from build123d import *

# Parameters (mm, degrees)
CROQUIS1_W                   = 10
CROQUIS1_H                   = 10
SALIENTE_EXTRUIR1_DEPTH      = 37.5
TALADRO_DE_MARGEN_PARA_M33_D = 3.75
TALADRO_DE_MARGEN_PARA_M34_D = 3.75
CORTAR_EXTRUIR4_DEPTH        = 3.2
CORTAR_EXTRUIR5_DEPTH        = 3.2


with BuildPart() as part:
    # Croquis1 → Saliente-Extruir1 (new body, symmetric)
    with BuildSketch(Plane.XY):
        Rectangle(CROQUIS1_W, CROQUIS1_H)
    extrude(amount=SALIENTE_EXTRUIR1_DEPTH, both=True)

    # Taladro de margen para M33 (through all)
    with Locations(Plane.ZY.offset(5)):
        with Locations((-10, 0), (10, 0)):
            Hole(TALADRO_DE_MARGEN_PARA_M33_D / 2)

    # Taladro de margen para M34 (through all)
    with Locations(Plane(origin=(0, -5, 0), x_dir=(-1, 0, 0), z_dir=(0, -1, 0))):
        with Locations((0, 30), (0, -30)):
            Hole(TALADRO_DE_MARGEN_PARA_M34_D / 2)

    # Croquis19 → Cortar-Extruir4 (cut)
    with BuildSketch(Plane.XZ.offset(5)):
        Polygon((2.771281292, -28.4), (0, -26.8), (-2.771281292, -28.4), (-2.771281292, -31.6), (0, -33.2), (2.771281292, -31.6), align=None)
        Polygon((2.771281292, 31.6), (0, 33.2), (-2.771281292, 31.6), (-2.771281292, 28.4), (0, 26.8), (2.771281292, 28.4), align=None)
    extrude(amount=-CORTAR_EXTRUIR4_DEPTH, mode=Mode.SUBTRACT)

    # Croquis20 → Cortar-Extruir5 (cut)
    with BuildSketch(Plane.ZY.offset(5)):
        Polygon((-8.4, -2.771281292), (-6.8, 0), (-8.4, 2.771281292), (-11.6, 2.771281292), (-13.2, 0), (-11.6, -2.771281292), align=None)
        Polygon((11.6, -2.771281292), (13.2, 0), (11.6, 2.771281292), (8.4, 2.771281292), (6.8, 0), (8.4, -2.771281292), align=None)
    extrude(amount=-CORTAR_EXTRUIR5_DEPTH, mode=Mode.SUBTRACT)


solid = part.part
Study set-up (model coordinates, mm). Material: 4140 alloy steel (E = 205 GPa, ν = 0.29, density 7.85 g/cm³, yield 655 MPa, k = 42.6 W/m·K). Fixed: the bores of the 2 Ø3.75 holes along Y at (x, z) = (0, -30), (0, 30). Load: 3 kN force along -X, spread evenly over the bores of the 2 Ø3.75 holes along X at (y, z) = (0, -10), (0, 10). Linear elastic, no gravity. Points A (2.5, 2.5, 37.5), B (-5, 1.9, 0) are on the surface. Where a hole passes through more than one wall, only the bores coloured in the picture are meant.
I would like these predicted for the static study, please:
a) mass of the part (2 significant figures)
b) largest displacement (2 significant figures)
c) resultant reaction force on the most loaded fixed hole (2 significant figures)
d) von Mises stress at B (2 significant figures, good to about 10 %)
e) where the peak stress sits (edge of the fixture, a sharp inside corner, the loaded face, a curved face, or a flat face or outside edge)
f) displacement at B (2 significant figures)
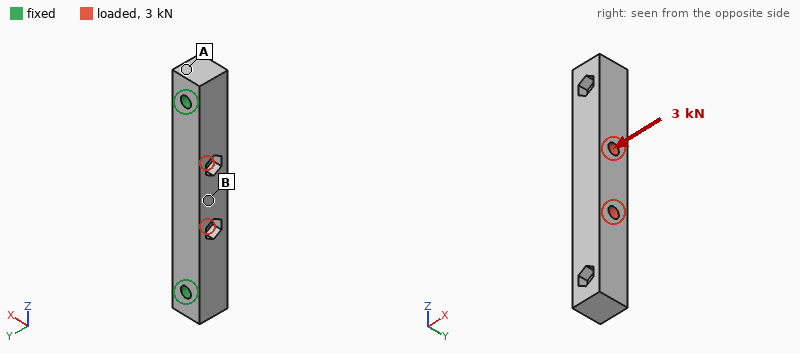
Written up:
54 g
30 µm
1.5 kN
62 MPa
edge of the fixture
29 µm
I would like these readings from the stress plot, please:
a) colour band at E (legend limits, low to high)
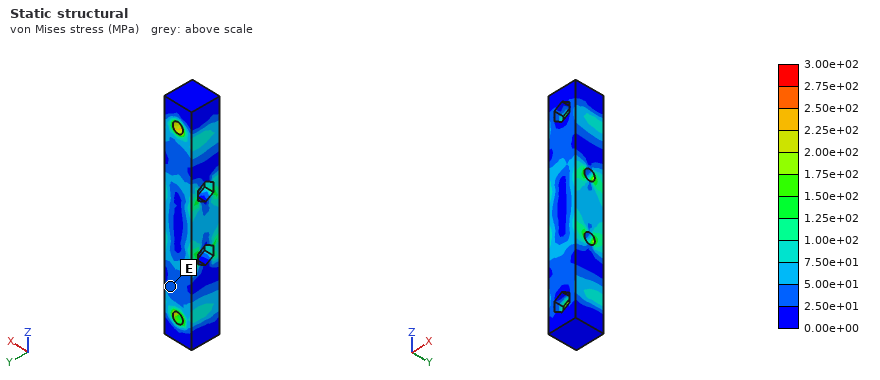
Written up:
2.50e+01 to 5.00e+01 MPa
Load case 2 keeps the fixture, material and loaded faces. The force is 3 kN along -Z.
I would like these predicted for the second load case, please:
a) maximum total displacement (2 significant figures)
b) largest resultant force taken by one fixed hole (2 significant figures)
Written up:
2.3 µm
1.5 kN
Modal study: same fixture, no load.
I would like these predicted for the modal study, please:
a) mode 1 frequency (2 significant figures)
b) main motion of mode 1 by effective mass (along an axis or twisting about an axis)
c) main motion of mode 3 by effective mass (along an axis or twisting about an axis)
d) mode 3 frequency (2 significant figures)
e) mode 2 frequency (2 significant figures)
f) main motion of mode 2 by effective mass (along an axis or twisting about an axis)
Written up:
10 kHz
along X
twisting about Z
22 kHz
11 kHz
along Y
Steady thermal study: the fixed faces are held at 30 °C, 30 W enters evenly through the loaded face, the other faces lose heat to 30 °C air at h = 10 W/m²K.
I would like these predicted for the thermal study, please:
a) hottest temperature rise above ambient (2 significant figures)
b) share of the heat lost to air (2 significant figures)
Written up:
83 K
4.1 %
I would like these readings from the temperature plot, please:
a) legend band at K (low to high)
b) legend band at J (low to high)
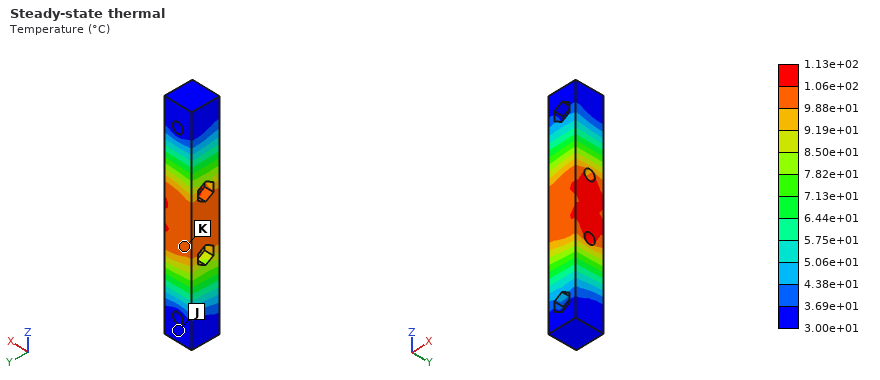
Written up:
9.88e+01 to 1.06e+02 °C
3.00e+01 to 3.69e+01 °C
